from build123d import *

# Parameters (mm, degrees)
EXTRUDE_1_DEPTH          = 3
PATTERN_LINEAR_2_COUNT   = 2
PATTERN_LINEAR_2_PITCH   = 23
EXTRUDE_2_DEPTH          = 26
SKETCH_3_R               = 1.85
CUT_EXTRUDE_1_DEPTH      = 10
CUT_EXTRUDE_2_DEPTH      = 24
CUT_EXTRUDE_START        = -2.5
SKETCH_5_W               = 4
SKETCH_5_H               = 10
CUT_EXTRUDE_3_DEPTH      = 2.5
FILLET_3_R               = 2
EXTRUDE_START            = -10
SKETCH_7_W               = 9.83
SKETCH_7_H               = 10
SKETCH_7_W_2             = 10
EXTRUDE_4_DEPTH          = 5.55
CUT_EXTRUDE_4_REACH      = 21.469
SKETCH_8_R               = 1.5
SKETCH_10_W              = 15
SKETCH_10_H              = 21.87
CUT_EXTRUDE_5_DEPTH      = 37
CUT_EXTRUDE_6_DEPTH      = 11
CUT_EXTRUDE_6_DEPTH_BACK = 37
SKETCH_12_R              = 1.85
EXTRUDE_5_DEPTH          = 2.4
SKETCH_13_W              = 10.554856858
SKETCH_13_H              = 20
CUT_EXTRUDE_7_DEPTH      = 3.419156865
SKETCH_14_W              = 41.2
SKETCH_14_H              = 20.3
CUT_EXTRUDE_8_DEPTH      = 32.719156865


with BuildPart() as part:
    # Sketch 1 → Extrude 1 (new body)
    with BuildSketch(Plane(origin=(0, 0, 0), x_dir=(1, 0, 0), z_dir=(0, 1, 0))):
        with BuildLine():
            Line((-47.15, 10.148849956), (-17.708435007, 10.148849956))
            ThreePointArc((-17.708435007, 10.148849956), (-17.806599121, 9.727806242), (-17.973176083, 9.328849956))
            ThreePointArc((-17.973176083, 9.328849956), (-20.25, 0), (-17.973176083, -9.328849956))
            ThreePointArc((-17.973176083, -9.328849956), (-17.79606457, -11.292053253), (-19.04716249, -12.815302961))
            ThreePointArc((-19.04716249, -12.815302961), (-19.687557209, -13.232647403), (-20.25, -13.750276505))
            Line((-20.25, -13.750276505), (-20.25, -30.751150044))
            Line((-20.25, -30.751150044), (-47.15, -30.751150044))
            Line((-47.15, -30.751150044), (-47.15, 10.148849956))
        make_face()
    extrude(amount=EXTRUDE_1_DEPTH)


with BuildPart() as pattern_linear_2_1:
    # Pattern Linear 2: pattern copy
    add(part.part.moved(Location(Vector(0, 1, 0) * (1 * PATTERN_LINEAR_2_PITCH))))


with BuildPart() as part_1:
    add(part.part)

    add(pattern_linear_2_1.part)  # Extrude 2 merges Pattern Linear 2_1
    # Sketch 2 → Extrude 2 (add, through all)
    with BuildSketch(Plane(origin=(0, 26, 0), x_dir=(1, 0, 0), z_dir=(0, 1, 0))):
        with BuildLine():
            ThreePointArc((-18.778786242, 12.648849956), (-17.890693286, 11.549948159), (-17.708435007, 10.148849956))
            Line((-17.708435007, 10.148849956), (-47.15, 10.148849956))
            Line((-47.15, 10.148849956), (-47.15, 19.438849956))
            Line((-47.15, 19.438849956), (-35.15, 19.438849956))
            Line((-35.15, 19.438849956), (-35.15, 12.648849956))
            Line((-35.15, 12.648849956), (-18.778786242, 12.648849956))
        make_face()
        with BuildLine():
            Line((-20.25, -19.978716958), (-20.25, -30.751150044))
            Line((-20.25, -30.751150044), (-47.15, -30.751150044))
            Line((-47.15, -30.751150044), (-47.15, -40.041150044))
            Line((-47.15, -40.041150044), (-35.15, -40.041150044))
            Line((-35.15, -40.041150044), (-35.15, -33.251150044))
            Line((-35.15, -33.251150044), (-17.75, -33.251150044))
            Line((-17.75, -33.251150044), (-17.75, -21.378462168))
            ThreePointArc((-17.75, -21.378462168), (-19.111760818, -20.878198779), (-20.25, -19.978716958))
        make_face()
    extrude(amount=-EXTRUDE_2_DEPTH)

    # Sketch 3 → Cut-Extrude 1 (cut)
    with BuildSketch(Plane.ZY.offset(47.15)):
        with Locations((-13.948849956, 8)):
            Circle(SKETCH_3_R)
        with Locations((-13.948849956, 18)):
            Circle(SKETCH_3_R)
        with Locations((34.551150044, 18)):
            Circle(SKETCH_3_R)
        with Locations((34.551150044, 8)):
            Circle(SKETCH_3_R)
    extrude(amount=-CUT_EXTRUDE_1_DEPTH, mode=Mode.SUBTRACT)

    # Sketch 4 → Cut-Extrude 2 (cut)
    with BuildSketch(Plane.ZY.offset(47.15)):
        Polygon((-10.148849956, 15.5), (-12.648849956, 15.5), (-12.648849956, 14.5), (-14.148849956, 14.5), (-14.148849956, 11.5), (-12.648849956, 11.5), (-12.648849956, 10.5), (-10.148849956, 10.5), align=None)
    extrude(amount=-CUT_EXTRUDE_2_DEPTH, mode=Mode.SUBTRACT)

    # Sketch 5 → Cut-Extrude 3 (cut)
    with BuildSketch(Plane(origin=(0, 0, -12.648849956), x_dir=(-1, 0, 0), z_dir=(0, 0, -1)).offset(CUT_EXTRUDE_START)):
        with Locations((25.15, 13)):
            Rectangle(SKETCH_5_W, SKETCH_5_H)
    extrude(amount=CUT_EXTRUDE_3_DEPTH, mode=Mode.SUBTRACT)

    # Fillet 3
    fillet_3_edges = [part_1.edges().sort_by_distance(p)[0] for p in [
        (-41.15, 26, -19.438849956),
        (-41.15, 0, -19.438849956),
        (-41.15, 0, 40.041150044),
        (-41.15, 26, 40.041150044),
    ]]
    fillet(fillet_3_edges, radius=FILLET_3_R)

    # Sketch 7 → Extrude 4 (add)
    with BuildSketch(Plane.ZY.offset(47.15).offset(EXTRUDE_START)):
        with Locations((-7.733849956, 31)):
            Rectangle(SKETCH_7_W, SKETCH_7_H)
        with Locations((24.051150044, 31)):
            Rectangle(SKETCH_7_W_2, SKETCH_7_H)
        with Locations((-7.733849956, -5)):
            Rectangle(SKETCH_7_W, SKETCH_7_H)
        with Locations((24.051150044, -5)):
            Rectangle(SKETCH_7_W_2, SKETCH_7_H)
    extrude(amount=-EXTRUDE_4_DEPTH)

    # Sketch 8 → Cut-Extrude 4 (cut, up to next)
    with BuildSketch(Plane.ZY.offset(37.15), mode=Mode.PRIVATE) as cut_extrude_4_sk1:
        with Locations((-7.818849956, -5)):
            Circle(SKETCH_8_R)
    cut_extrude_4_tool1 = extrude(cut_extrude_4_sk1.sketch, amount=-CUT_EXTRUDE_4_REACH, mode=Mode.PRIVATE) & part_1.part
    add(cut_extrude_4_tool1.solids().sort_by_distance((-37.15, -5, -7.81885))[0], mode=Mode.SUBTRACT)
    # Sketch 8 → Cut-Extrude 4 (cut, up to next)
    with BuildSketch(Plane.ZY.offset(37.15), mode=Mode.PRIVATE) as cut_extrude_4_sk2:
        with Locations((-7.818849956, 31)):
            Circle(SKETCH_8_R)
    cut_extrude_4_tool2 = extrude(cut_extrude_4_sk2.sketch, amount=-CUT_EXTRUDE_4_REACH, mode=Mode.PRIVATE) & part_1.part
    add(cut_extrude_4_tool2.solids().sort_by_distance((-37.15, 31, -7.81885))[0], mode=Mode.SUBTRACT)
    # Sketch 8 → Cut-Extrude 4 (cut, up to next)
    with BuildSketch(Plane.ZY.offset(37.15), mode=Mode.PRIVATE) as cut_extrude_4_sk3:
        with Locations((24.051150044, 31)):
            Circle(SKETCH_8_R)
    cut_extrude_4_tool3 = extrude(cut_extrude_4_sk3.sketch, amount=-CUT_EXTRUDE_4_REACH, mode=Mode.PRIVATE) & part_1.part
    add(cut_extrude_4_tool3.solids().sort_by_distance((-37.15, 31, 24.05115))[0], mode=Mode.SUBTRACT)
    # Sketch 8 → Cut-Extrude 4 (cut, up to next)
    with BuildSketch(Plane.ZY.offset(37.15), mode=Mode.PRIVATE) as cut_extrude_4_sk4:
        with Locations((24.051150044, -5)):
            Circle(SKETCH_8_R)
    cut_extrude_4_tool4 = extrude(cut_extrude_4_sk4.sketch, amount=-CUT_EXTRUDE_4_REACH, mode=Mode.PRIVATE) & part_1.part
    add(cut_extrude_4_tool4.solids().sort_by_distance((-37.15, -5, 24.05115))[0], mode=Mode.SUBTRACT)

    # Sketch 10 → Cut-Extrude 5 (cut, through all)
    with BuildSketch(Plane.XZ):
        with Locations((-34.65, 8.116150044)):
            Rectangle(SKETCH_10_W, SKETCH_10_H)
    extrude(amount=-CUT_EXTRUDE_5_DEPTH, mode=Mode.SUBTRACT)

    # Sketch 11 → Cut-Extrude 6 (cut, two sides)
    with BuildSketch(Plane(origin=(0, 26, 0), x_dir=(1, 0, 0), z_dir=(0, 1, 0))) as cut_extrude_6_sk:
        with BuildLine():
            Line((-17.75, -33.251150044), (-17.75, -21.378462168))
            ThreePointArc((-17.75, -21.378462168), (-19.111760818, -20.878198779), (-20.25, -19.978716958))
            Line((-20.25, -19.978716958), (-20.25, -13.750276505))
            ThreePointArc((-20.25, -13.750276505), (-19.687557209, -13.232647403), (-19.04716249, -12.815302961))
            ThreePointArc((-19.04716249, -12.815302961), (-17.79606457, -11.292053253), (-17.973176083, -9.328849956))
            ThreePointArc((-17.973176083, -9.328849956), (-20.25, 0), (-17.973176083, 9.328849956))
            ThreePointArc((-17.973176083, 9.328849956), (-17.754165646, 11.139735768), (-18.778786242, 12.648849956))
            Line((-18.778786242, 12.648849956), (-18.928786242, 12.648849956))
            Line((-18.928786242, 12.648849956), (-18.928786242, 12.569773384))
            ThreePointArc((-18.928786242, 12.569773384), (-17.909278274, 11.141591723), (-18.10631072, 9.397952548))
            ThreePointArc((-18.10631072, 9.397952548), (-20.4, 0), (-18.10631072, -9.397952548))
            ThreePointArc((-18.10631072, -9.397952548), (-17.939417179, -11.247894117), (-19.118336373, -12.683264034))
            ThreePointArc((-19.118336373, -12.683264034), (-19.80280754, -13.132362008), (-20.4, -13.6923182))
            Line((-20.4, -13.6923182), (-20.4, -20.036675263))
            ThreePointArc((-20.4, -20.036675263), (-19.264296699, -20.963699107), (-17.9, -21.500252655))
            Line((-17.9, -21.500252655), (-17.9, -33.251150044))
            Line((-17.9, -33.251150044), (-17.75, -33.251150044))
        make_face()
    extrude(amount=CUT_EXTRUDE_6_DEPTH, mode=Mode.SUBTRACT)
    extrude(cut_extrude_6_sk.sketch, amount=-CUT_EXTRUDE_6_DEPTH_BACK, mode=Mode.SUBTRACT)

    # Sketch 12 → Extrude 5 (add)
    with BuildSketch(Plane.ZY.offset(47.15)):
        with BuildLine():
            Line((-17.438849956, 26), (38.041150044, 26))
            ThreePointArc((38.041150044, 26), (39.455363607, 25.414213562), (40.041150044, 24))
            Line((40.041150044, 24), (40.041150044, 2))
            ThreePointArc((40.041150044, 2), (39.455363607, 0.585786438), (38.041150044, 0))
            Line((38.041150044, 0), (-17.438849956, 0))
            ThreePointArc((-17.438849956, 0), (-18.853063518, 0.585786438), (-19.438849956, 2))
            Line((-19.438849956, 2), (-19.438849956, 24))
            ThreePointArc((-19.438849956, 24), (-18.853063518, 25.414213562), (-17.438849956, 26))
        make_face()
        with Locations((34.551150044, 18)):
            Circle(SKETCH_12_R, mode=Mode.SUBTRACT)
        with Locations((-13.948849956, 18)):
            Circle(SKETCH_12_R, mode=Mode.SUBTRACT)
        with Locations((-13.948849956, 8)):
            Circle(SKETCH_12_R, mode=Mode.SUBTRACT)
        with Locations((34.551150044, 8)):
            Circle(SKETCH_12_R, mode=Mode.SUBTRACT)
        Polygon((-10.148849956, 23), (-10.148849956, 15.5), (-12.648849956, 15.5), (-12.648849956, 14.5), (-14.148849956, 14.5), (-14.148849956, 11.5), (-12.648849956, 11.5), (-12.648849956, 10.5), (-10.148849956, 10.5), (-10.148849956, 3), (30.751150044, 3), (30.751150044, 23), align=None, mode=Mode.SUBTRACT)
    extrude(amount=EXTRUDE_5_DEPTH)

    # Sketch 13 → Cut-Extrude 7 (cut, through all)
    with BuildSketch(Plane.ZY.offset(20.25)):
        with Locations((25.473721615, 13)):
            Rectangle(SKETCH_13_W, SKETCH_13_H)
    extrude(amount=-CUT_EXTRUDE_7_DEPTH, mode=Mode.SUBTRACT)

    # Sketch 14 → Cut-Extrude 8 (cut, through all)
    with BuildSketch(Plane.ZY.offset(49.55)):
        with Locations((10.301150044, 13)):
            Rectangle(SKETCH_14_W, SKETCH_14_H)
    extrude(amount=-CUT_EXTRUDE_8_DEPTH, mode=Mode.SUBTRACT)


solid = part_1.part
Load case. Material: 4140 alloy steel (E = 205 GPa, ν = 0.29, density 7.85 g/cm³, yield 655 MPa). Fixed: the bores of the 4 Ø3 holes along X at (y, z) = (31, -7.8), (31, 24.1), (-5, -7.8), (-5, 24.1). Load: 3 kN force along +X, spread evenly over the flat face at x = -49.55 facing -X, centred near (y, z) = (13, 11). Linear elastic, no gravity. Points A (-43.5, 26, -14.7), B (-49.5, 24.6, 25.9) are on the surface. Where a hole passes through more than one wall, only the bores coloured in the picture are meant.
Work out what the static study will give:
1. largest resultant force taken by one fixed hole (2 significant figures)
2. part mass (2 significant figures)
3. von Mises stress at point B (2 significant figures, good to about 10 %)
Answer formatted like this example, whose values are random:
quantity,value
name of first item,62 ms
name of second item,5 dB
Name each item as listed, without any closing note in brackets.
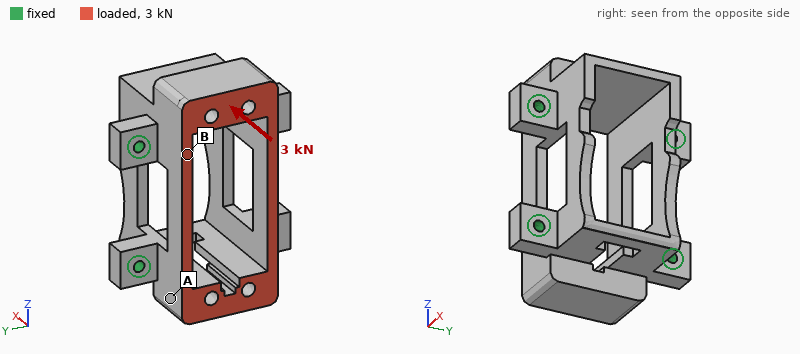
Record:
quantity,value
largest resultant force taken by one fixed hole,840 N
part mass,120 g
von Mises stress at point B,29 MPa
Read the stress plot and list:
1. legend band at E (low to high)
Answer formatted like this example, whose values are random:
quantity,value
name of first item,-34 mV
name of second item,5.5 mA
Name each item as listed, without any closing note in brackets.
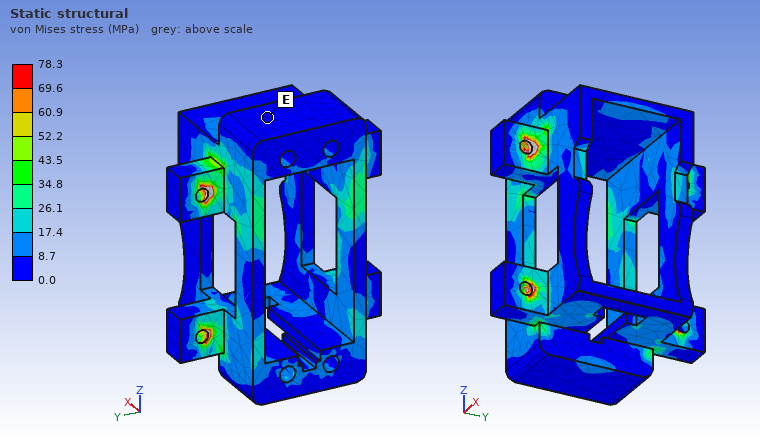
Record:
quantity,value
legend band at E,0.0 to 8.7 MPa
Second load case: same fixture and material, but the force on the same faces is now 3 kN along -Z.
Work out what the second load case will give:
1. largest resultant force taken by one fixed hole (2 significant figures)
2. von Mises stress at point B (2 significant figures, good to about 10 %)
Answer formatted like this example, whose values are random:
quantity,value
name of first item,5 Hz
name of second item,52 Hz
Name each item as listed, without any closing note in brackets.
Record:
quantity,value
largest resultant force taken by one fixed hole,1.0 kN
von Mises stress at point B,50 MPa
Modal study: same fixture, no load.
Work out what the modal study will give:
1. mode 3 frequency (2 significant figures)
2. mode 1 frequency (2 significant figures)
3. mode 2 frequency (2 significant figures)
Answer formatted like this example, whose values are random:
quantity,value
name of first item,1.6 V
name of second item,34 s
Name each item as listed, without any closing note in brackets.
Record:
quantity,value
mode 3 frequency,9900 Hz
mode 1 frequency,8100 Hz
mode 2 frequency,9300 Hz
